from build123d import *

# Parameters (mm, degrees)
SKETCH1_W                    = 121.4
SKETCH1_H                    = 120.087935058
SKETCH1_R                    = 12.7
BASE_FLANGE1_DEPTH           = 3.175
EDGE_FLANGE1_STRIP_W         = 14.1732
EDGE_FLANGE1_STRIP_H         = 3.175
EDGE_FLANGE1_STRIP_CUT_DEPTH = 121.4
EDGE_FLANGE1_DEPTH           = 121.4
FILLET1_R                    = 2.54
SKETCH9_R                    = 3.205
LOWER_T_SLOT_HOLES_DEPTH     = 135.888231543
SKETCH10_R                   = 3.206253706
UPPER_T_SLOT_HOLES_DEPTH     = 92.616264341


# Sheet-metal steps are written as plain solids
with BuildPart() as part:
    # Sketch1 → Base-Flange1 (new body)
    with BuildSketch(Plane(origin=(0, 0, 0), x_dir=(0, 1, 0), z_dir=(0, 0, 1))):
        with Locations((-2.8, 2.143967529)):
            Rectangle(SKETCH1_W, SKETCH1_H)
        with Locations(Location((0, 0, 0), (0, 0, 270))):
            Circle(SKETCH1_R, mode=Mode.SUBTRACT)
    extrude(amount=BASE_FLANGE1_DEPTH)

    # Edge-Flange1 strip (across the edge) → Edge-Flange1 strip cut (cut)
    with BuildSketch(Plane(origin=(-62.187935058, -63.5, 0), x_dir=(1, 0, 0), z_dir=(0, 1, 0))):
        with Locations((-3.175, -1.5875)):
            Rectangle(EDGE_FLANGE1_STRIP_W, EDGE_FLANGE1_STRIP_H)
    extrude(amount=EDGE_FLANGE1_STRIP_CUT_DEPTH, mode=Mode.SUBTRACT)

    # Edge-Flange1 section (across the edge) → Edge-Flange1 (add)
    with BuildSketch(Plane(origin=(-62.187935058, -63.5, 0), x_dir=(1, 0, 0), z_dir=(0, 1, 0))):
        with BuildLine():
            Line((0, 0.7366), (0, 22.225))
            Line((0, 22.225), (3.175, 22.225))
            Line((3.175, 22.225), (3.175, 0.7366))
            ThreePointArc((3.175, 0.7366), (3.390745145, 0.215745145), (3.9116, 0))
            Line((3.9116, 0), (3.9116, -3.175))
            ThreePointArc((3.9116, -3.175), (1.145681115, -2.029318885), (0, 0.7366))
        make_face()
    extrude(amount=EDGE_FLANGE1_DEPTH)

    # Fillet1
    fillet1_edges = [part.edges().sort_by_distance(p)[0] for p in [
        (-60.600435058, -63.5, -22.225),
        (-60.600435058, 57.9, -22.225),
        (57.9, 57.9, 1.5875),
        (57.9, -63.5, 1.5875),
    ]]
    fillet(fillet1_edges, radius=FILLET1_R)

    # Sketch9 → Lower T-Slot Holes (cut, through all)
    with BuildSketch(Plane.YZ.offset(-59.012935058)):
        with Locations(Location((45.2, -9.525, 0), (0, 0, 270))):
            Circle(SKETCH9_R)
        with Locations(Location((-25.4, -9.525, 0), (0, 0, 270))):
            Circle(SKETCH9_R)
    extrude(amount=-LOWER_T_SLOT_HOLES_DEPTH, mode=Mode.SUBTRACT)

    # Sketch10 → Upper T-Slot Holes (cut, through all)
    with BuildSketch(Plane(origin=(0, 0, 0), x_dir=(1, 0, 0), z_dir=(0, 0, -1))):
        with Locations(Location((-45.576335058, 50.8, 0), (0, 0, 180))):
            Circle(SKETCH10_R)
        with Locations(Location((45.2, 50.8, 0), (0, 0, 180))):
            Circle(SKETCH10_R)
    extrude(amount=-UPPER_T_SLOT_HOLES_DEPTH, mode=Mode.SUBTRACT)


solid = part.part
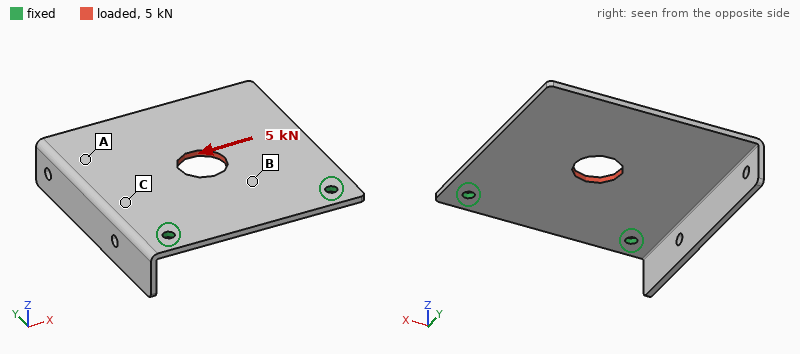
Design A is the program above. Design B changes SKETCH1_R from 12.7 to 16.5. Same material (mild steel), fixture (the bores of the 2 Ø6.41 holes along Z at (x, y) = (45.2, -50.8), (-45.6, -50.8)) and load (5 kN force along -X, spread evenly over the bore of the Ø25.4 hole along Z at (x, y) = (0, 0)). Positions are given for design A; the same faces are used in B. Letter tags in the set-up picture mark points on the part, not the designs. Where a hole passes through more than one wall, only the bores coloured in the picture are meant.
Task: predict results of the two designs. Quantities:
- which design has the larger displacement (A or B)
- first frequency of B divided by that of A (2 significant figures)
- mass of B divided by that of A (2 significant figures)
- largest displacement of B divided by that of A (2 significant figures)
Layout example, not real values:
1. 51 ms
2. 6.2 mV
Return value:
1. B
2. 1.0
3. 0.98
4. 1.1
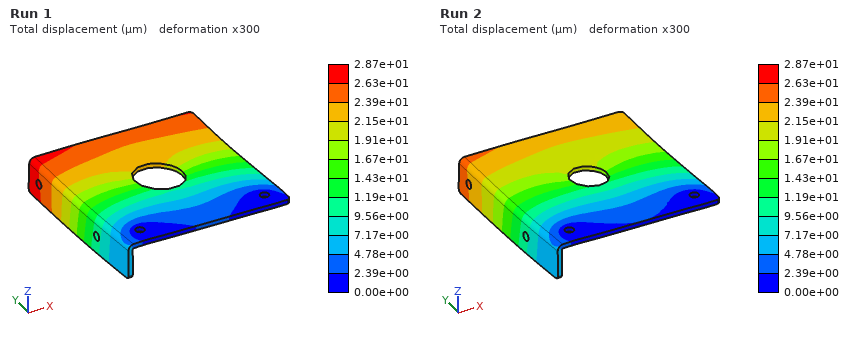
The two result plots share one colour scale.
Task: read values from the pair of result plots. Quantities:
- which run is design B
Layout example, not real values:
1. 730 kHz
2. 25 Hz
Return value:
1. Run 1
